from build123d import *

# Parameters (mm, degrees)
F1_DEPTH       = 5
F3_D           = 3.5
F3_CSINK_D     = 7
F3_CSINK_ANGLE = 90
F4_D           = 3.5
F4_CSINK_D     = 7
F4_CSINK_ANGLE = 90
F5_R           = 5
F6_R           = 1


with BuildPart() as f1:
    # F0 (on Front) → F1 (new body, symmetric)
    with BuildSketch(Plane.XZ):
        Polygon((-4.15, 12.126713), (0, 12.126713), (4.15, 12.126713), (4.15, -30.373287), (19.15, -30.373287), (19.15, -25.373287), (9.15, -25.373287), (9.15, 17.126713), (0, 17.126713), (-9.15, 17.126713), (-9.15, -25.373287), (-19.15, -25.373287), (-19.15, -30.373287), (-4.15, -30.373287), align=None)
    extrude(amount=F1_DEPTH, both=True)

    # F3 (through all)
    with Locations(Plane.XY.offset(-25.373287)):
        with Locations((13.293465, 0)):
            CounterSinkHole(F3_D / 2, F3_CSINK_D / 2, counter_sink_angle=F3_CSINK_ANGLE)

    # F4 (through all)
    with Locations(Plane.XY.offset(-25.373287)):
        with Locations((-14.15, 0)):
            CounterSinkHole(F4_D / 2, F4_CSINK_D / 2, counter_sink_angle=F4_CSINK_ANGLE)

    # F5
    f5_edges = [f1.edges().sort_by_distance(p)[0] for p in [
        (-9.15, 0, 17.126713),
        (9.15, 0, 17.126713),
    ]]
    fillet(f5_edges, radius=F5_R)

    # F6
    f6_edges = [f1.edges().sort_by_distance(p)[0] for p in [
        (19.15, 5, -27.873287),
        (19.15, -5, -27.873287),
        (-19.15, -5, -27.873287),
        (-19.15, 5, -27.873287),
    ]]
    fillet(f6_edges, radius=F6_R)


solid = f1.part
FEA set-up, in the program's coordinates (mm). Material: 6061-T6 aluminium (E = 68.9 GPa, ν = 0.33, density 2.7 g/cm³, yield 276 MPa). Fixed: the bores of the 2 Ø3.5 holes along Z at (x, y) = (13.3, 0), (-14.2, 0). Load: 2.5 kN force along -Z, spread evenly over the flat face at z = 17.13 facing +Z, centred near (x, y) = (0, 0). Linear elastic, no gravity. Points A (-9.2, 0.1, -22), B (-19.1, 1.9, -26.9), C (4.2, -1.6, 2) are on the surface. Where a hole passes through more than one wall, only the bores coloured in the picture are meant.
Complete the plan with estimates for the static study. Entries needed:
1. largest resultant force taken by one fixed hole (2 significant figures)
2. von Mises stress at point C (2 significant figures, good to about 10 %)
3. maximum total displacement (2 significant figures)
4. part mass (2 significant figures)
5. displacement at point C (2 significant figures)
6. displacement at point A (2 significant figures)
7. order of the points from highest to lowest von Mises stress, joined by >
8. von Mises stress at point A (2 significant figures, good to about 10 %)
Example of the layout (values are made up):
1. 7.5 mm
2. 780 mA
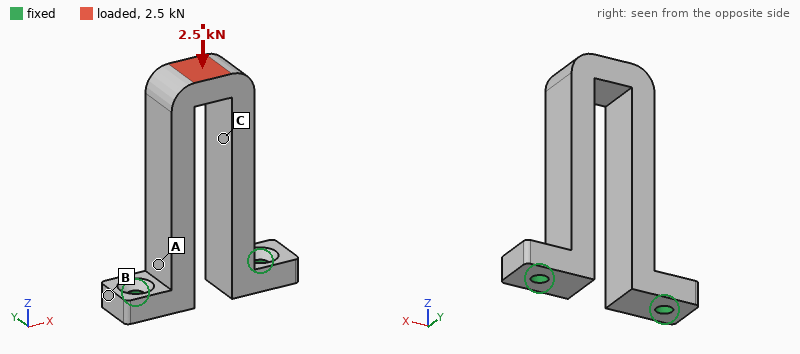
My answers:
1. 1.3 kN
2. 48 MPa
3. 48 µm
4. 16 g
5. 28 µm
6. 28 µm
7. A > C > B
8. 81 MPa
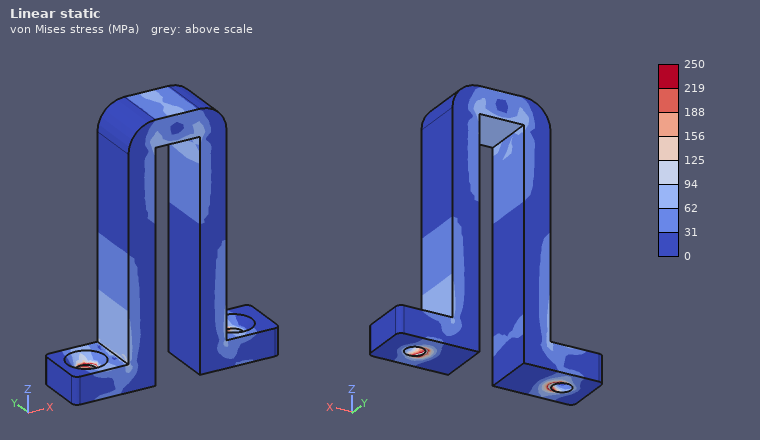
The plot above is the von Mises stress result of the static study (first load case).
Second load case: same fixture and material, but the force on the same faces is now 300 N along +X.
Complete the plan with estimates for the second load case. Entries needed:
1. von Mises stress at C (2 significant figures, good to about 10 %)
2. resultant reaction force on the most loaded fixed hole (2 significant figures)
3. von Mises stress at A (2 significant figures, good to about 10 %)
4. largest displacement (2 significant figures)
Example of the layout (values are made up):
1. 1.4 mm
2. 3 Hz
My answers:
1. 40 MPa
2. 550 N
3. 67 MPa
4. 0.17 mm
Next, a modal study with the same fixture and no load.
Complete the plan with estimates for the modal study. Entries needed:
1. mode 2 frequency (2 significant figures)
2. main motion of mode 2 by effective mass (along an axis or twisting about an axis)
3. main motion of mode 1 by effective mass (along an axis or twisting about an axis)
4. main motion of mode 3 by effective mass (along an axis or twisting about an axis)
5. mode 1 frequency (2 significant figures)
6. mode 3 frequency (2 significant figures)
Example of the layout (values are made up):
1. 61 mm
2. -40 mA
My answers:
1. 2700 Hz
2. along X
3. along Y
4. twisting about Z
5. 2000 Hz
6. 6300 Hz
